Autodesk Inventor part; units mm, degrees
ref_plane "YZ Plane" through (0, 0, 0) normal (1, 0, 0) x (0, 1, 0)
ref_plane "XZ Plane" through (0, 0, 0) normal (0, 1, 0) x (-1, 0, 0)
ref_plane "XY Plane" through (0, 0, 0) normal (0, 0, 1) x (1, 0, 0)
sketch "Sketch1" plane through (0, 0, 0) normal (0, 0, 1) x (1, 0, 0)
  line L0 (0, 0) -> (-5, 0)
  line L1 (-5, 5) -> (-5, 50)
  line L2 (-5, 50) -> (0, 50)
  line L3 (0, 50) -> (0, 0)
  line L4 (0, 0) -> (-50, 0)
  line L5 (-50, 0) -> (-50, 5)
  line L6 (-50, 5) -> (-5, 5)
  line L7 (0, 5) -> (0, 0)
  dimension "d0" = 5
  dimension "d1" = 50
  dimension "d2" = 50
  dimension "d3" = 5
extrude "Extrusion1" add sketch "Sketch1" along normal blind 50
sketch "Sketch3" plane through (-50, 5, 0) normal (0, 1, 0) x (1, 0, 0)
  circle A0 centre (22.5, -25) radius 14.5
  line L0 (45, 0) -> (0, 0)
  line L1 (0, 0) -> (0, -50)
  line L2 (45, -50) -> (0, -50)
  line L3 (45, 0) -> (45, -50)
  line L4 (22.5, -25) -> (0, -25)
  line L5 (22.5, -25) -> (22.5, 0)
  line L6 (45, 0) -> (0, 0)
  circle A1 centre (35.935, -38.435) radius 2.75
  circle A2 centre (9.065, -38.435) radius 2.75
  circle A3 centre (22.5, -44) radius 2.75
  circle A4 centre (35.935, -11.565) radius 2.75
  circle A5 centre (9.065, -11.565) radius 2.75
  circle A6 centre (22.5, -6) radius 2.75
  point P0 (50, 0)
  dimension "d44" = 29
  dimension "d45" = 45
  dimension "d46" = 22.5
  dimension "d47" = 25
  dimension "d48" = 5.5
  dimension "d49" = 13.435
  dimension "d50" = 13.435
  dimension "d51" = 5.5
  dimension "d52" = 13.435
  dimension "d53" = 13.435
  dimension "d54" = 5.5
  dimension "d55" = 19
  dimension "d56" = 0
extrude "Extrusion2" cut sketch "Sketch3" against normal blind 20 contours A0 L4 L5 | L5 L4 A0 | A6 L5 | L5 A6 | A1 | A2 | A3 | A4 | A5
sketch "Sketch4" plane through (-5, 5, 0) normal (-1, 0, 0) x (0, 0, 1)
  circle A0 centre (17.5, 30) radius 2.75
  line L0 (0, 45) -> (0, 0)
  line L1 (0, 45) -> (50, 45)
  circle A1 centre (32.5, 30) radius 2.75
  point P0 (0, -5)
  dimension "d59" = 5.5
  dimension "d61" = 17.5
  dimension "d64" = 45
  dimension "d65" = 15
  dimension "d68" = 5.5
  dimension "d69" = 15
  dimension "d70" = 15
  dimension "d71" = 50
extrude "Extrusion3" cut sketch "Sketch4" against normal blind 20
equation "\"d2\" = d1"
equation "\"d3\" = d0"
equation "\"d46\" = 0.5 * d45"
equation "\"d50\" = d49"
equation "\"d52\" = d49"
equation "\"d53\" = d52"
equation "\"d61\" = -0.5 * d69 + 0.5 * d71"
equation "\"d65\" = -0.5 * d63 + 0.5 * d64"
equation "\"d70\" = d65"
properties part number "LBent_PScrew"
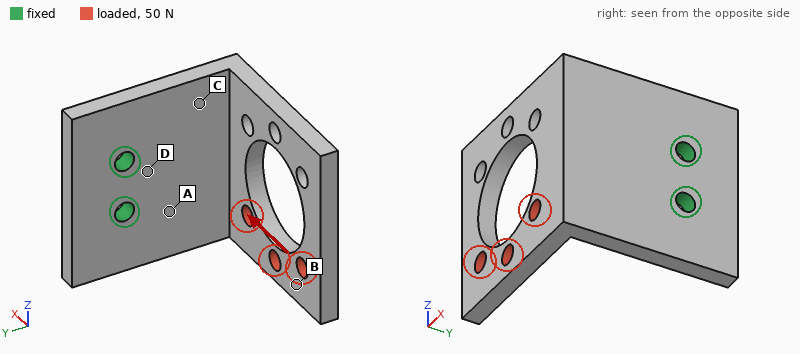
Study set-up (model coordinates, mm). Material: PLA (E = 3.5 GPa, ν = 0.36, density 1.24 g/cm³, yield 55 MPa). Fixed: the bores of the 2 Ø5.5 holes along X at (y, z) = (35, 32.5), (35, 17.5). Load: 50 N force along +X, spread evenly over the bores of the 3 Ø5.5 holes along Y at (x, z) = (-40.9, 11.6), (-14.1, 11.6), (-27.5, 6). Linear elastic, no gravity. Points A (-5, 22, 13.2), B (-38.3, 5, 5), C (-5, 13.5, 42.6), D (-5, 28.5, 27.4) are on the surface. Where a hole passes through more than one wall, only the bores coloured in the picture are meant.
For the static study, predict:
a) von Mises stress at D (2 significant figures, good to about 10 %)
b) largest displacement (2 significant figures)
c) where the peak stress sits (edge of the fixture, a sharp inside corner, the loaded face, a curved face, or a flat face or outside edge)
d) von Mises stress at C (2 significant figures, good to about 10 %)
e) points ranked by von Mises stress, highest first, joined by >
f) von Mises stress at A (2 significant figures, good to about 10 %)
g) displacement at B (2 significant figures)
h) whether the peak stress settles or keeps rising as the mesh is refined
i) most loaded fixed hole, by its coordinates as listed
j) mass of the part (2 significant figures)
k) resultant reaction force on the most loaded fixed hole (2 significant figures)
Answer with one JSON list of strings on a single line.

["6.1 MPa", "0.91 mm", "edge of the fixture", "3.3 MPa", "D > A > C > B", "5.0 MPa", "0.70 mm", "keeps rising", "(35, 17.5)", "24 g", "54 N"]
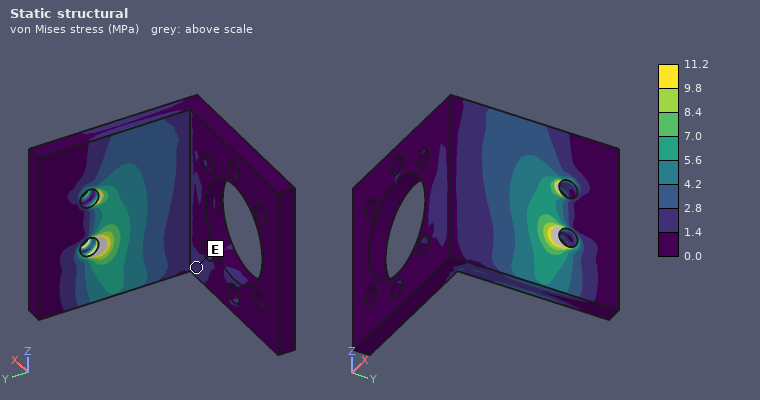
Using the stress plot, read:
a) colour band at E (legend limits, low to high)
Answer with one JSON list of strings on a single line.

["1.4 to 2.8 MPa"]
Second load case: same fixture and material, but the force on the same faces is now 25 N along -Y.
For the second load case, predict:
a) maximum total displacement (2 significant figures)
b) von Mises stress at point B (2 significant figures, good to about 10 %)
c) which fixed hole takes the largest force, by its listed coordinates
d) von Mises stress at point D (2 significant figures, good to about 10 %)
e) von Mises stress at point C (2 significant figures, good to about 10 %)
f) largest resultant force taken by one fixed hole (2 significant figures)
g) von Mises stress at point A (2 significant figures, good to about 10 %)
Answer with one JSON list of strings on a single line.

["0.98 mm", "0.78 MPa", "(35, 17.5)", "3.0 MPa", "2.3 MPa", "33 N", "3.2 MPa"]
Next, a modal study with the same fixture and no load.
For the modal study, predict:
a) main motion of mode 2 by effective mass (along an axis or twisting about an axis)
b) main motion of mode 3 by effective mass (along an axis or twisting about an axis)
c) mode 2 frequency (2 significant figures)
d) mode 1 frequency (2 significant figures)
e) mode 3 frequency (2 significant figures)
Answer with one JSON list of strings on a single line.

["along Z", "along X", "520 Hz", "310 Hz", "800 Hz"]
